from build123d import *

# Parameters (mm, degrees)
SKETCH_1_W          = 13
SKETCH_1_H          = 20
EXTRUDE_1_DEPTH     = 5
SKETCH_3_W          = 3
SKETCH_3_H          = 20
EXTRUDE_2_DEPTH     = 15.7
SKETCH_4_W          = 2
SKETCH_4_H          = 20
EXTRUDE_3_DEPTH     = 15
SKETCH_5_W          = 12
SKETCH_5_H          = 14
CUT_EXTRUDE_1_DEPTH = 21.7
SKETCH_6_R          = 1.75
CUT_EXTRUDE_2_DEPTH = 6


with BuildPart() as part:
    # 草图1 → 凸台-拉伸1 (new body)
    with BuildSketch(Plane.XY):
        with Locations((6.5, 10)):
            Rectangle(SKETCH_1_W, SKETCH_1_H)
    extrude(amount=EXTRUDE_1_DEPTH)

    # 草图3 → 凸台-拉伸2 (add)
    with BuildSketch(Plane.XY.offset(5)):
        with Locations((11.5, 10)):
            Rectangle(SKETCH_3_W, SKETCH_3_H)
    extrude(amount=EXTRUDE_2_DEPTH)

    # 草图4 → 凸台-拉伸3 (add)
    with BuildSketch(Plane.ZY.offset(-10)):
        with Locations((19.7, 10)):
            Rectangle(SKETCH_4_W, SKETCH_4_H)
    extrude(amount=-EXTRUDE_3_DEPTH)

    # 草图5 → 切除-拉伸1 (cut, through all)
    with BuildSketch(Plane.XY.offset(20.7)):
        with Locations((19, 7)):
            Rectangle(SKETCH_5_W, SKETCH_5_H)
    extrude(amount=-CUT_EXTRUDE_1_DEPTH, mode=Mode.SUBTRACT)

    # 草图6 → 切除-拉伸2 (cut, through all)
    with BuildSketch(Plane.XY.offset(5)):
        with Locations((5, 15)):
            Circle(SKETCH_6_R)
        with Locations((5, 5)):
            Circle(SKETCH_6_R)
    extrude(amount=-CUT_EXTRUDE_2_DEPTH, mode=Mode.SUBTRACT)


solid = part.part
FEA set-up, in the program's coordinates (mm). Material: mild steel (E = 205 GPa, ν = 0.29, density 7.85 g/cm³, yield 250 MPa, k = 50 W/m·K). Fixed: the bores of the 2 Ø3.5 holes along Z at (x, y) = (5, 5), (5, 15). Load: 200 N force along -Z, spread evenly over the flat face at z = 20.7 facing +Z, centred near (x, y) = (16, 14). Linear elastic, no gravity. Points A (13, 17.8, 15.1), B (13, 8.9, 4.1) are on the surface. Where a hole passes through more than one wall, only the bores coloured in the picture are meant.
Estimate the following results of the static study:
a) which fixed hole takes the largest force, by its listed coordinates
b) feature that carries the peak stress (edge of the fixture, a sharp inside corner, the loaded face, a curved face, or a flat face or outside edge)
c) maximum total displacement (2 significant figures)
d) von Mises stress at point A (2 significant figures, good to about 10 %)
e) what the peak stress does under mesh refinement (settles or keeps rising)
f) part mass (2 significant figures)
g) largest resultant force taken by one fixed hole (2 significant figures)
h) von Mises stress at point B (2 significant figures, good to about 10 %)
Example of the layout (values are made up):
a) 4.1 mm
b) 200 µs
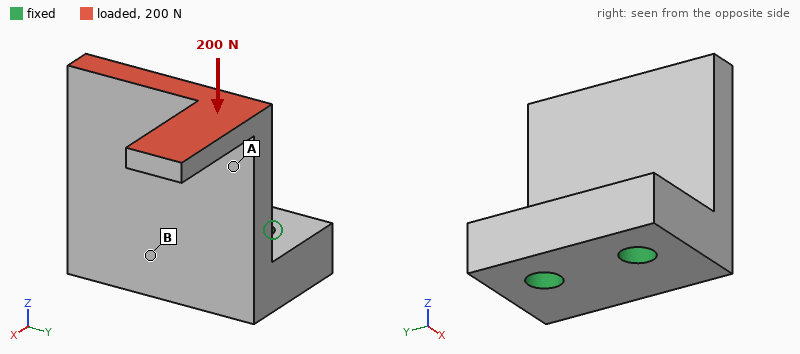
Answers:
a) (5, 15)
b) a sharp inside corner
c) 73 µm
d) 54 MPa
e) keeps rising
f) 18 g
g) 150 N
h) 22 MPa
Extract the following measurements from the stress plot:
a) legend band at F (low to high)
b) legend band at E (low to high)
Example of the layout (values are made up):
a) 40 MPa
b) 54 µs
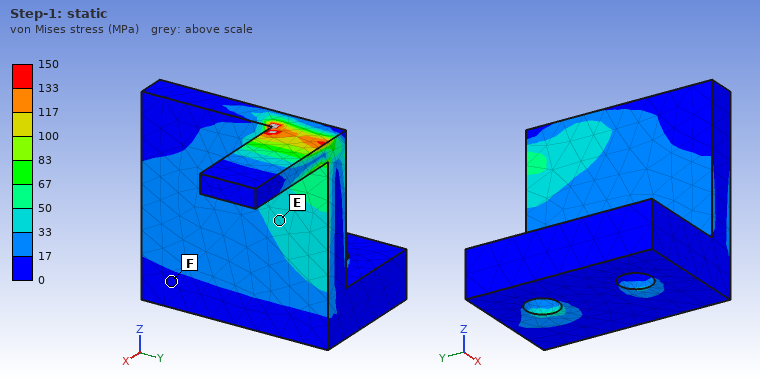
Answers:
a) 0 to 17 MPa
b) 33 to 50 MPa
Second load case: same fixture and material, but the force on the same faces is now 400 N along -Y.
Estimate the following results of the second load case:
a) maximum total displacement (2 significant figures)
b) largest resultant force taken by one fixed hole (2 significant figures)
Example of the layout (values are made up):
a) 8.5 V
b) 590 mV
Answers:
a) 57 µm
b) 640 N
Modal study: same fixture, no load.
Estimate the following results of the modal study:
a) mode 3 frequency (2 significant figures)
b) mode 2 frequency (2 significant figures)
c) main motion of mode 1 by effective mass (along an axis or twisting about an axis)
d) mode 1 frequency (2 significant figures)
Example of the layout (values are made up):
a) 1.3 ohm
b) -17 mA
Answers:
a) 10 kHz
b) 9700 Hz
c) along X
d) 5400 Hz
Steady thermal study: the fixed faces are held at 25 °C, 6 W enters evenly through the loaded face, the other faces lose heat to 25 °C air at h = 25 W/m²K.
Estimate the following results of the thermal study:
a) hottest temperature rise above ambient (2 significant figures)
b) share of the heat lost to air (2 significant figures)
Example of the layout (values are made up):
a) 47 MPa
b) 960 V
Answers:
a) 77 K
b) 11 %
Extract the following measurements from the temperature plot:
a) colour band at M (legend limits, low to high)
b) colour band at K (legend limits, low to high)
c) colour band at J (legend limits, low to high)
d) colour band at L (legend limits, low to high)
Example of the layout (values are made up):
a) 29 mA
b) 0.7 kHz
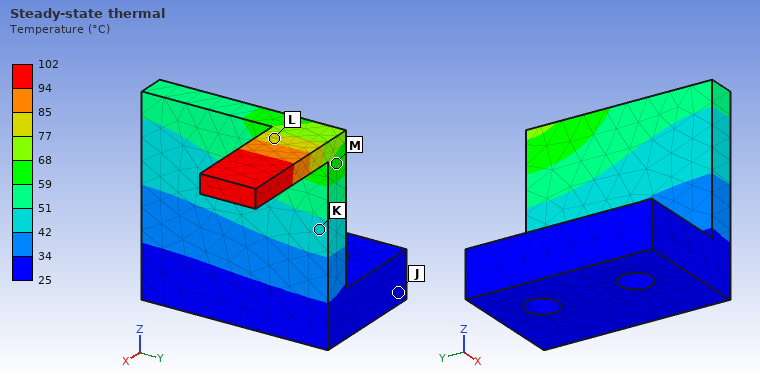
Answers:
a) 59 to 68 °C
b) 42 to 51 °C
c) 25 to 34 °C
d) 77 to 85 °C
